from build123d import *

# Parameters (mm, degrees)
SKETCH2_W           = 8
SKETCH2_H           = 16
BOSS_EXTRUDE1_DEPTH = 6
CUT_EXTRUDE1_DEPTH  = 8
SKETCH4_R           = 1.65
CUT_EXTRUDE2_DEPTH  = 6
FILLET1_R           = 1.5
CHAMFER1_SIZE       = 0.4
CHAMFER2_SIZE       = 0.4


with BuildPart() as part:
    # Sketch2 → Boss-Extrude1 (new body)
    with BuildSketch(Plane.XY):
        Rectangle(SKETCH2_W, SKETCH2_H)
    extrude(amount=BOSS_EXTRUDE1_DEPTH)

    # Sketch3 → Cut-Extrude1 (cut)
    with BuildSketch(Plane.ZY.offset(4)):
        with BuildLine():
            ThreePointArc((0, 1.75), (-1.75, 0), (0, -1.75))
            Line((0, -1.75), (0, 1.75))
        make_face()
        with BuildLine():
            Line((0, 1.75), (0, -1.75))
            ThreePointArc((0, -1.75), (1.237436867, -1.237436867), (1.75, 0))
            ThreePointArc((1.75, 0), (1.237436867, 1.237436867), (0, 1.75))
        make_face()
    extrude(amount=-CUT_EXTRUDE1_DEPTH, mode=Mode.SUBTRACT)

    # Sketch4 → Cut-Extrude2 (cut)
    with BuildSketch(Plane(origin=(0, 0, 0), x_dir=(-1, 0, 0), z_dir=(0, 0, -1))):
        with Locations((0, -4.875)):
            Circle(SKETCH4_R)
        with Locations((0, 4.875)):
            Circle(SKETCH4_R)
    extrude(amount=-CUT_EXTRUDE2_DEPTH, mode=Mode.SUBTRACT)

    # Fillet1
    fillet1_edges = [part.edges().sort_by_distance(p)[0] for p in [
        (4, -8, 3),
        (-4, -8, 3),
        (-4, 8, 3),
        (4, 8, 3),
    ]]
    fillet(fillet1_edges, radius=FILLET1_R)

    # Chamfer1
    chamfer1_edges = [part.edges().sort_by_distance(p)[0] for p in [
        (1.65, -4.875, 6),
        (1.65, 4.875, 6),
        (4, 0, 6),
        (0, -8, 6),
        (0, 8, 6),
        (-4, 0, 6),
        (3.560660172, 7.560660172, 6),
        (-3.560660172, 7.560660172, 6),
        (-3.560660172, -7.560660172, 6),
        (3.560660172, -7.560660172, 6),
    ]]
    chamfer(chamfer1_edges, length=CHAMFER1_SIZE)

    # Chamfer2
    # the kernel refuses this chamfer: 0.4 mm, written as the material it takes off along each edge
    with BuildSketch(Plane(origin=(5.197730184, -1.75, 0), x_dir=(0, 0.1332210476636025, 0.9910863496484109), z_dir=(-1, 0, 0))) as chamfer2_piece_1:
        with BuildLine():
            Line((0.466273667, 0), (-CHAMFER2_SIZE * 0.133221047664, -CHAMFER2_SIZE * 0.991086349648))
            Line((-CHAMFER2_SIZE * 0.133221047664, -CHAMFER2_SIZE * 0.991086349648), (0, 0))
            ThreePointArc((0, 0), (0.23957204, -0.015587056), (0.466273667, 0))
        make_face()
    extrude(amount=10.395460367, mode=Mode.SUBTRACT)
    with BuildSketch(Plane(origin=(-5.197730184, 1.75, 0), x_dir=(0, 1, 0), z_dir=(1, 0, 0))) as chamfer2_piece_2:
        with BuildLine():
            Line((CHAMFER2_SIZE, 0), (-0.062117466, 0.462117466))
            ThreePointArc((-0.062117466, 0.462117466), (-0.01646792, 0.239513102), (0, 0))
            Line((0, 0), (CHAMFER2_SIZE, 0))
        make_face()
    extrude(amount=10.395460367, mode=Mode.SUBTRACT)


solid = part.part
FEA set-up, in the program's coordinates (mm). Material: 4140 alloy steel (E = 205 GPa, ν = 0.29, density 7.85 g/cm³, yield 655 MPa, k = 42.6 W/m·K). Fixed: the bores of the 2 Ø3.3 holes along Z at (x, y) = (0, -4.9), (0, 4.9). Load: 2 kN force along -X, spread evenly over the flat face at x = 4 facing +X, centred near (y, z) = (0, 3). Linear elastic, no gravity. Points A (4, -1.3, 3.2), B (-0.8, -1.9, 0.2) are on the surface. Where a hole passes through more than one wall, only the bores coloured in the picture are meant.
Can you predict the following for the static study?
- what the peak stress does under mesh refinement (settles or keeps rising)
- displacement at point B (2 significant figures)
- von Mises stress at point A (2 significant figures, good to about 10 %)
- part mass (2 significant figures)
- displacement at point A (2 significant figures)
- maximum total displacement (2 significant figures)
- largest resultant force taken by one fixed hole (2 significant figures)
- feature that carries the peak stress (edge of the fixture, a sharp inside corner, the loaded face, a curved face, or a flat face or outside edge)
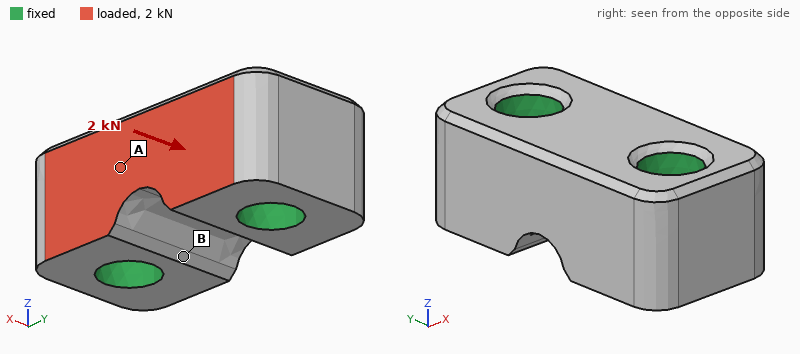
keeps rising
0.18 µm
22 MPa
4.8 g
0.71 µm
0.75 µm
1.0 kN
edge of the fixture
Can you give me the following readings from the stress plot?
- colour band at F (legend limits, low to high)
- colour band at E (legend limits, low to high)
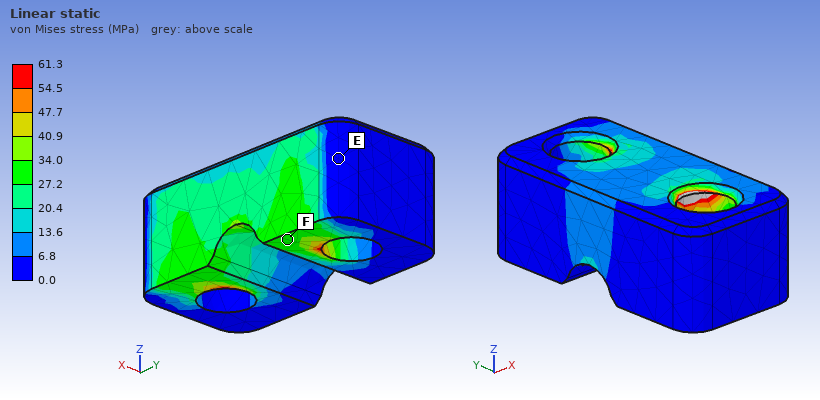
27.2 to 34.0 MPa
0.0 to 6.8 MPa
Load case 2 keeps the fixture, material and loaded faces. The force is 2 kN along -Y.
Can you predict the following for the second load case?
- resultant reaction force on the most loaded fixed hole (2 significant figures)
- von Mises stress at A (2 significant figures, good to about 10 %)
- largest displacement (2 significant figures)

1.1 kN
52 MPa
1.6 µm
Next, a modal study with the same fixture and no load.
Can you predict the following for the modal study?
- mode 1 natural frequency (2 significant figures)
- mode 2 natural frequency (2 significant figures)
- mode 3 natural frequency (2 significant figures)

160 kHz
170 kHz
190 kHz
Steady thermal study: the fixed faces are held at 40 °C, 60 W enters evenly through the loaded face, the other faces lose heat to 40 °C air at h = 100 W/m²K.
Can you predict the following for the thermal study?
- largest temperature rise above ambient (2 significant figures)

72 K
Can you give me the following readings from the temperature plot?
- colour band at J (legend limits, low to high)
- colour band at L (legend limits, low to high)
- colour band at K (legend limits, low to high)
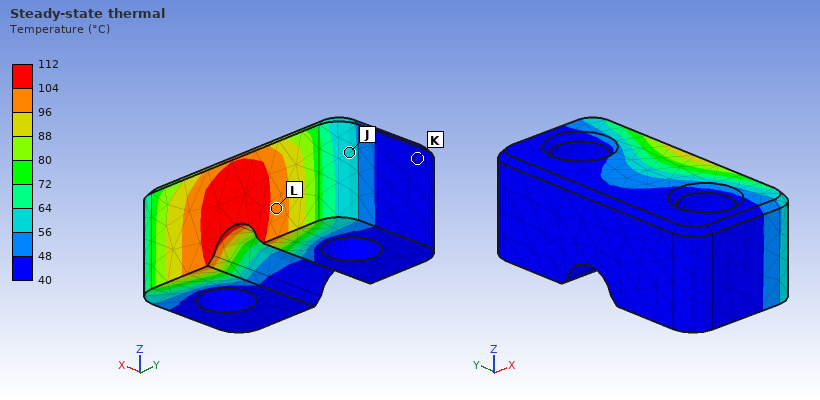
56 to 64 °C
96 to 104 °C
40 to 48 °C
